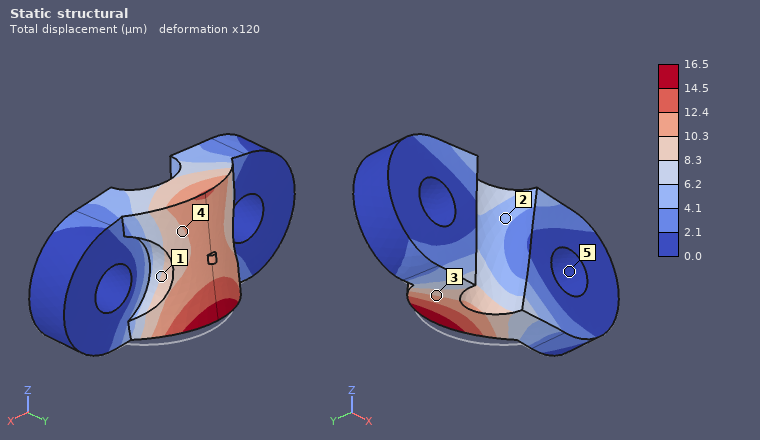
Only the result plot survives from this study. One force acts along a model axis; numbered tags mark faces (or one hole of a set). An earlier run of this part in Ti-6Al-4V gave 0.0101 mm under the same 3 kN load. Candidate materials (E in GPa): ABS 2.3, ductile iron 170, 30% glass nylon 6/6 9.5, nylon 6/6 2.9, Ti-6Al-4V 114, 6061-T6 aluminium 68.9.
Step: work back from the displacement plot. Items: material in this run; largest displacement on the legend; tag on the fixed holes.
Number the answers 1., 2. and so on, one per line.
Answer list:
1. 6061-T6 aluminium
2. 16.5 µm
3. 5
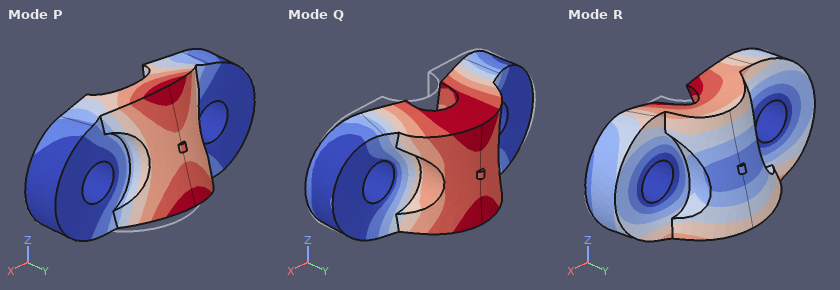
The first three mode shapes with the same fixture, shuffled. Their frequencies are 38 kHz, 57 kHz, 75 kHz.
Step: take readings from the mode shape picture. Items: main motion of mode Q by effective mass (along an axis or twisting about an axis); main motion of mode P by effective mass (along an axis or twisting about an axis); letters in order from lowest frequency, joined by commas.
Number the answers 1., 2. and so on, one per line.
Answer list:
1. along Y
2. along Z
3. P, Q, R
